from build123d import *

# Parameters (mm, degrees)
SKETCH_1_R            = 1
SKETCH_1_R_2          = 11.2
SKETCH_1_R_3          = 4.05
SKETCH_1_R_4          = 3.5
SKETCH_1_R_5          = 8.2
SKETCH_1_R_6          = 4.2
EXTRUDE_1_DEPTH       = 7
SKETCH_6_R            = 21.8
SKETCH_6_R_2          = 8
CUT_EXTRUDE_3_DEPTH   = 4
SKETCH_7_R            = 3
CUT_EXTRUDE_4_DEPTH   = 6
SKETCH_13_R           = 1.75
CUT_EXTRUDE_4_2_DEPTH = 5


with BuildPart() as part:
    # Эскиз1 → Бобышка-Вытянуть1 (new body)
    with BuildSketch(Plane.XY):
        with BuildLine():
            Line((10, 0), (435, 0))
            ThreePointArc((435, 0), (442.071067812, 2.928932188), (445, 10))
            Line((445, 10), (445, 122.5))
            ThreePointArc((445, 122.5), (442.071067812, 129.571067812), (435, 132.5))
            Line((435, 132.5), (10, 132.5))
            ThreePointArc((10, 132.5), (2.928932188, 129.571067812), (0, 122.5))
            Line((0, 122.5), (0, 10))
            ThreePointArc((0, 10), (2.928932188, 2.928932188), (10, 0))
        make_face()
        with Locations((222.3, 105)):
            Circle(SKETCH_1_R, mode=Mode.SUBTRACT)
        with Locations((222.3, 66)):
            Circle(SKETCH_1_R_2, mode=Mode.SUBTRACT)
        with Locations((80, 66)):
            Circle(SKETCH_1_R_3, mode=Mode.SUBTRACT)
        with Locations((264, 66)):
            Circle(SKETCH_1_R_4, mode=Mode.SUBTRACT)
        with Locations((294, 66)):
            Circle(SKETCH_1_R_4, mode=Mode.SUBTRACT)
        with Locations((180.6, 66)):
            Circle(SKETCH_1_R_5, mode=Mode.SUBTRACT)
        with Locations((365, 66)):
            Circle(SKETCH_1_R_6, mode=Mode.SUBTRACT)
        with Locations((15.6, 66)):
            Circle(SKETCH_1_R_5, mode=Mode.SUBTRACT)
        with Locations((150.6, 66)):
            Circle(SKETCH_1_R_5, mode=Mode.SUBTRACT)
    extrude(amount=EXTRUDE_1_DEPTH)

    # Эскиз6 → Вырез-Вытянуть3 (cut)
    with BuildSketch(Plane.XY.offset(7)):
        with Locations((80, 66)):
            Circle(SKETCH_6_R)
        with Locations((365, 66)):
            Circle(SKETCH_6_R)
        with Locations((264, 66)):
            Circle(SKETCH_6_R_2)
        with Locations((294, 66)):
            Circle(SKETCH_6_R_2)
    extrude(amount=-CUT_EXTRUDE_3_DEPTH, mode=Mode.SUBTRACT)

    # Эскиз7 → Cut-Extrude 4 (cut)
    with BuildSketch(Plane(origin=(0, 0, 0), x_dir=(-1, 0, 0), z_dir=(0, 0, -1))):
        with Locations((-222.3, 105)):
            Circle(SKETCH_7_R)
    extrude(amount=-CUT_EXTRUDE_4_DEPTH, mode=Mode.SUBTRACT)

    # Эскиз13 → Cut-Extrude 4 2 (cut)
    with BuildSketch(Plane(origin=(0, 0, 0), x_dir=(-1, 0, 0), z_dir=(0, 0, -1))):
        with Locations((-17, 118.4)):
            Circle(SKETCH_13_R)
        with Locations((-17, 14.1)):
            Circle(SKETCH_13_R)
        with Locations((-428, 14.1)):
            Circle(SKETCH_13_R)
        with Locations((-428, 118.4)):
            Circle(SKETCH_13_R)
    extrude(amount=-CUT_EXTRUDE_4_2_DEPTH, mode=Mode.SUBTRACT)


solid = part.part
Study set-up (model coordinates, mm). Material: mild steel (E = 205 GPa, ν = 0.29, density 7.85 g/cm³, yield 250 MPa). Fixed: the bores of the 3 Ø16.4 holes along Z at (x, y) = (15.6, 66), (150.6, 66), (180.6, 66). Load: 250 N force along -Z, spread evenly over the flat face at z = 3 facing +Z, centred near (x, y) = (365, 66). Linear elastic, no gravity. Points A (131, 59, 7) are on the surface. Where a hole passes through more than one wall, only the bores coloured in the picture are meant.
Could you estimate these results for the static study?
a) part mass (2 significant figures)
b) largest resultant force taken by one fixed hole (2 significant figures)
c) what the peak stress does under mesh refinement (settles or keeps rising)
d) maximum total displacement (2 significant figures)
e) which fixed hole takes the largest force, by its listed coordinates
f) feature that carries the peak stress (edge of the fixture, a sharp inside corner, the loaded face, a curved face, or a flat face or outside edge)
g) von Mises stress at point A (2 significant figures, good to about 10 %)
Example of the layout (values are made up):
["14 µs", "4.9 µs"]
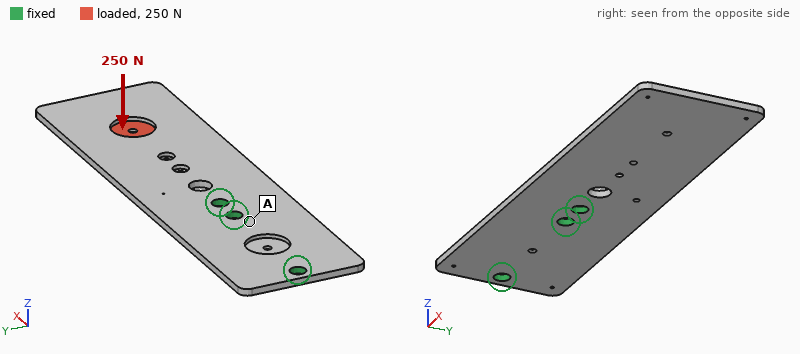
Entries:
["3.1 kg", "790 N", "keeps rising", "1.2 mm", "(180.6, 66)", "edge of the fixture", "5.7 MPa"]
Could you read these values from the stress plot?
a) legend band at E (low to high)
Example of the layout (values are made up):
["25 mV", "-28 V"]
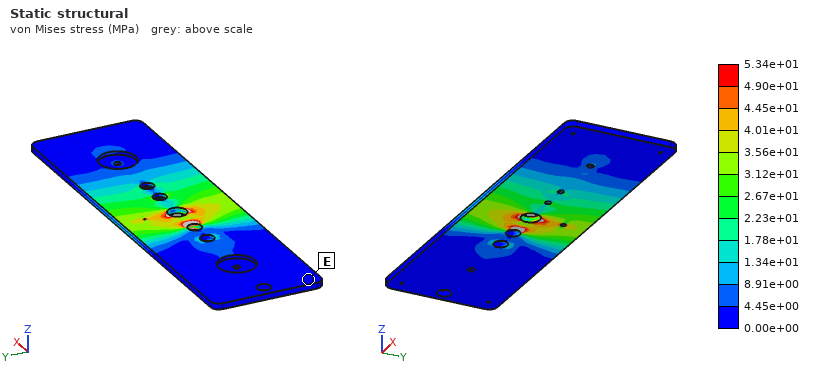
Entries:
["0.00e+00 to 4.45e+00 MPa"]
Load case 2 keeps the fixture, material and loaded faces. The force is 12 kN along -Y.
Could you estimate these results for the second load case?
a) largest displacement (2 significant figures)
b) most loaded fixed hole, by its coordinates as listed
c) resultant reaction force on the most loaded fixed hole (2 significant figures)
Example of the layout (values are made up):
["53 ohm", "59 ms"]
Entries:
["0.36 mm", "(180.6, 66)", "31 kN"]
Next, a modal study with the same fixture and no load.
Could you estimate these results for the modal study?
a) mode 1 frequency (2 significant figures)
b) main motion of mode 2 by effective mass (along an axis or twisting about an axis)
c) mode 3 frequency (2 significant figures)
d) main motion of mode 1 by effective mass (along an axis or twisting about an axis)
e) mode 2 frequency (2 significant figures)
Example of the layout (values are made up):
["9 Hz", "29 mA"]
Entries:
["81 Hz", "twisting about X", "490 Hz", "along Z", "310 Hz"]
